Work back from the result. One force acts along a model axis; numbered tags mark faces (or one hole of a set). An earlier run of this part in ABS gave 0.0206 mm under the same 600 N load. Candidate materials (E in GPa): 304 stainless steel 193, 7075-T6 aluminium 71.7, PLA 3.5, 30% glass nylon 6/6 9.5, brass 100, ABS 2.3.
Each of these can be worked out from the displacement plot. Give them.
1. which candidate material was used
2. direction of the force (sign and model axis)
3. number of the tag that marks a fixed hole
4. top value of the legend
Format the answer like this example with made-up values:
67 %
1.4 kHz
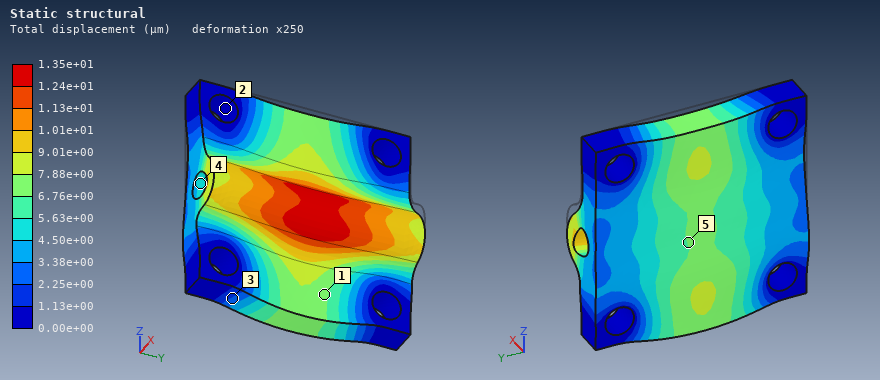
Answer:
PLA
-Z
2
1.35e+01 µm
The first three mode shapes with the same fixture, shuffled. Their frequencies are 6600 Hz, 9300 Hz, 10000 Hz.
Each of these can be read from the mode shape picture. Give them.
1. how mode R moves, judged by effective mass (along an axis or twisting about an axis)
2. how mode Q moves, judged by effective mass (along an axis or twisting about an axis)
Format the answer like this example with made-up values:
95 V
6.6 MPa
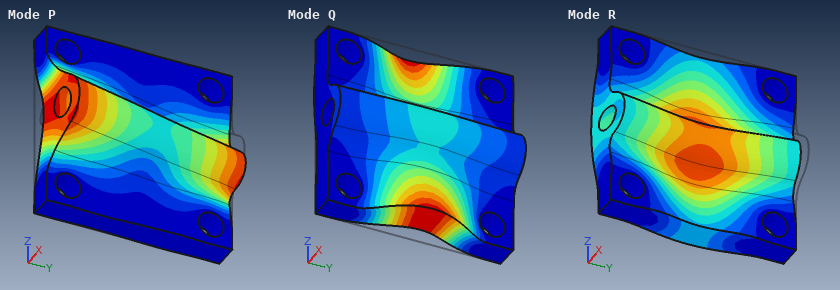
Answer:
along X
twisting about Y
